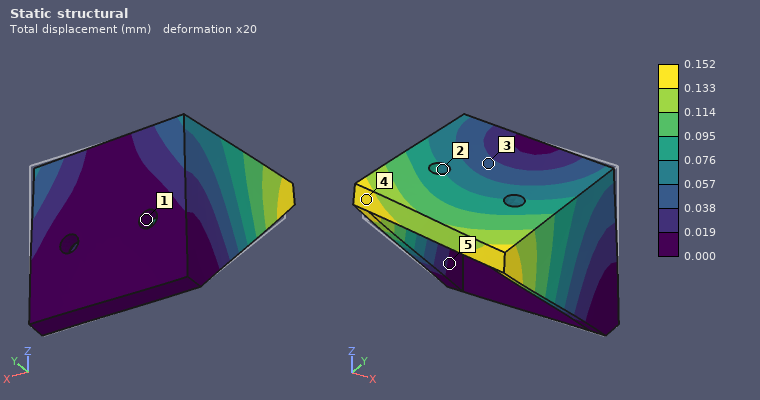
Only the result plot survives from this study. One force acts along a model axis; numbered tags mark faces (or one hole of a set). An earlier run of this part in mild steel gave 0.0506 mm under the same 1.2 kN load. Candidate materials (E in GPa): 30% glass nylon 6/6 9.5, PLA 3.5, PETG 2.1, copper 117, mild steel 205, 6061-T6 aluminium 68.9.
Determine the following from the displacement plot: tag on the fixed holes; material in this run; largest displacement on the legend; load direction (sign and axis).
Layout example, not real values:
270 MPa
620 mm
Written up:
1
6061-T6 aluminium
0.152 mm
-X
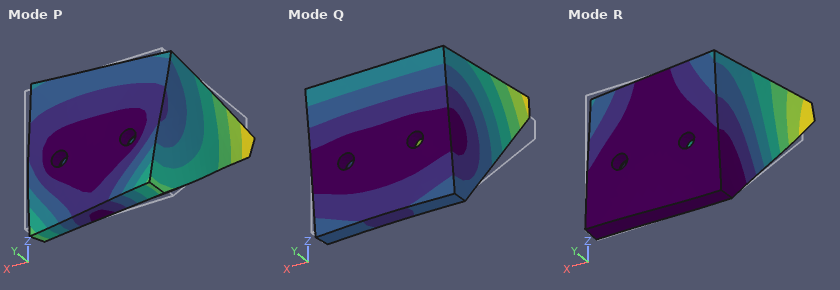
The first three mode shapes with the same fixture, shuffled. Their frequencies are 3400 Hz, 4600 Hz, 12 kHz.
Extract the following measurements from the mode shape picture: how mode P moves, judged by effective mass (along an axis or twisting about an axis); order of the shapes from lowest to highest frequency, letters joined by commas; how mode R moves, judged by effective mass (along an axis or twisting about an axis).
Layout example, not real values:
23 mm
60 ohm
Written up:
along X
Q, R, P
along X
